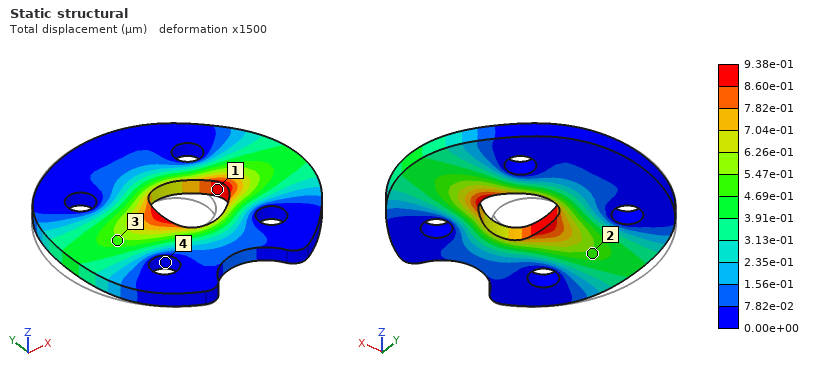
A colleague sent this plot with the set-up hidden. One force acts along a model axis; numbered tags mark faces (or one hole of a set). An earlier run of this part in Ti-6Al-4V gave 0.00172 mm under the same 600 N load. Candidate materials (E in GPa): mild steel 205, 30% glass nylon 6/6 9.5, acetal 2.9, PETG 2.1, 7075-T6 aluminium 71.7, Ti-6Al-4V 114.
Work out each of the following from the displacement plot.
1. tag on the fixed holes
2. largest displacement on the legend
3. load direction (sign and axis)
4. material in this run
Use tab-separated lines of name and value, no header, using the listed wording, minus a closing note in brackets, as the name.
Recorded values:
tag on the fixed holes	4
largest displacement on the legend	9.38e-01 µm
load direction	+X
material in this run	mild steel
